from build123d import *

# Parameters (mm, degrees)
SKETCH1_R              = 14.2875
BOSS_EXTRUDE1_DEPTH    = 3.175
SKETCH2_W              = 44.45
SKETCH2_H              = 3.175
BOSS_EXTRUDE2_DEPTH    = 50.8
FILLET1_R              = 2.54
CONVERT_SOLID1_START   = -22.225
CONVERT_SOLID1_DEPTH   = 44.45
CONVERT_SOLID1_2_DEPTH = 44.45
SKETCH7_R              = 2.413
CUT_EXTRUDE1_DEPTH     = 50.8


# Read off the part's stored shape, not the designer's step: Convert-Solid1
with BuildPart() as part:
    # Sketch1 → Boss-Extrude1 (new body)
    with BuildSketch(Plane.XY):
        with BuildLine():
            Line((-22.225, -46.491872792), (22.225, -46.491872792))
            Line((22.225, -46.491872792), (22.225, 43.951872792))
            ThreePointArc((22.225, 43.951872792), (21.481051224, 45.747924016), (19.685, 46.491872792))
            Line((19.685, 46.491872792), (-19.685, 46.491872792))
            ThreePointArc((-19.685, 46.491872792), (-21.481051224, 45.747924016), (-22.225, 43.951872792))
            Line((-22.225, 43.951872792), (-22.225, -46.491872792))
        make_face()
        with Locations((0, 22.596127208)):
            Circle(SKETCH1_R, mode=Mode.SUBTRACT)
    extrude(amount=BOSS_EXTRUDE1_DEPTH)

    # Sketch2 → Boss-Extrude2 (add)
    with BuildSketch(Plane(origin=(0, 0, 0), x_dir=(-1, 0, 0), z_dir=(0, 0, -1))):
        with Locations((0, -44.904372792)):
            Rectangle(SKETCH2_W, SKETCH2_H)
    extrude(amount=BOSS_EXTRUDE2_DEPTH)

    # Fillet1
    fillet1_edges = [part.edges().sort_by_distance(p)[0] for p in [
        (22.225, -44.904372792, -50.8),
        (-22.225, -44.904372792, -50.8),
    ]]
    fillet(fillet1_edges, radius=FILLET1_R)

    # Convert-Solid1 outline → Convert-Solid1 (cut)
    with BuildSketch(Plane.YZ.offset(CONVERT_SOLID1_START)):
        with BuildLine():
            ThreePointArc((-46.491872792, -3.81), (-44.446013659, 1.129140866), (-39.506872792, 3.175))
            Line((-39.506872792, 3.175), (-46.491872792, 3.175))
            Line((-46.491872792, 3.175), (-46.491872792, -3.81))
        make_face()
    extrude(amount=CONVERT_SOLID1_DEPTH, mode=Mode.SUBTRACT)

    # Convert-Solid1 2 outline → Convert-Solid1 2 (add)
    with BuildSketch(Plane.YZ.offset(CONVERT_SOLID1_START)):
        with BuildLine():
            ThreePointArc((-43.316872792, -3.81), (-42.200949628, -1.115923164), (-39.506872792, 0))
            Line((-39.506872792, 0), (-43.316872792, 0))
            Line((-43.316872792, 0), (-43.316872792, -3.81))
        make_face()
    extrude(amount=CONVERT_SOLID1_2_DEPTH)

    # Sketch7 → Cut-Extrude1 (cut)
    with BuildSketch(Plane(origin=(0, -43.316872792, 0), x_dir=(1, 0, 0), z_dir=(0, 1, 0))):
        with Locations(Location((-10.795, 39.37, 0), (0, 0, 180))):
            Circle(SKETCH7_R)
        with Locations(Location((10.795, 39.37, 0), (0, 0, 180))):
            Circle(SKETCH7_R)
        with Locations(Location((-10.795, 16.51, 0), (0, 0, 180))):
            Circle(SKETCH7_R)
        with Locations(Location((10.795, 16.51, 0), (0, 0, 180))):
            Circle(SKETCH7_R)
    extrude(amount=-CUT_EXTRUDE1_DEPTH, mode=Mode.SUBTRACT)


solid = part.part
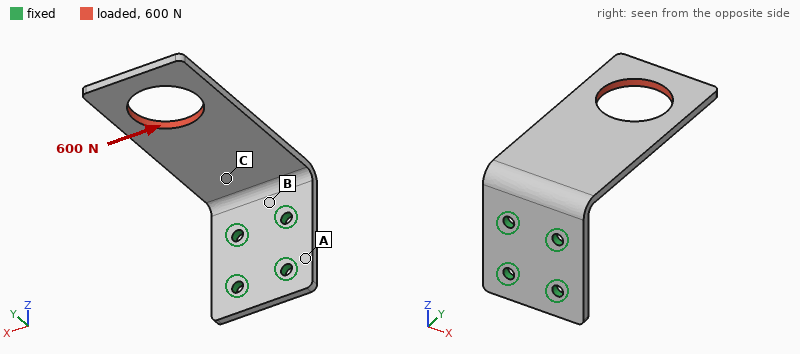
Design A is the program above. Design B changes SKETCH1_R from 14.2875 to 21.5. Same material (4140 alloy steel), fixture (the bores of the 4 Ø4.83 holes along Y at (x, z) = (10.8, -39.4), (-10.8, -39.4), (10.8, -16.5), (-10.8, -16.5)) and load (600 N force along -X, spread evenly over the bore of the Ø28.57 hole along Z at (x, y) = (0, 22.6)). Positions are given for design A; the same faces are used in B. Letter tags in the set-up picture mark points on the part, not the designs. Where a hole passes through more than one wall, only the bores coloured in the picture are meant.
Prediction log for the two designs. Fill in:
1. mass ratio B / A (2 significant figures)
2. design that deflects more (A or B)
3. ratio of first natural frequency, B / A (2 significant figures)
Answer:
0.85
B
1.2
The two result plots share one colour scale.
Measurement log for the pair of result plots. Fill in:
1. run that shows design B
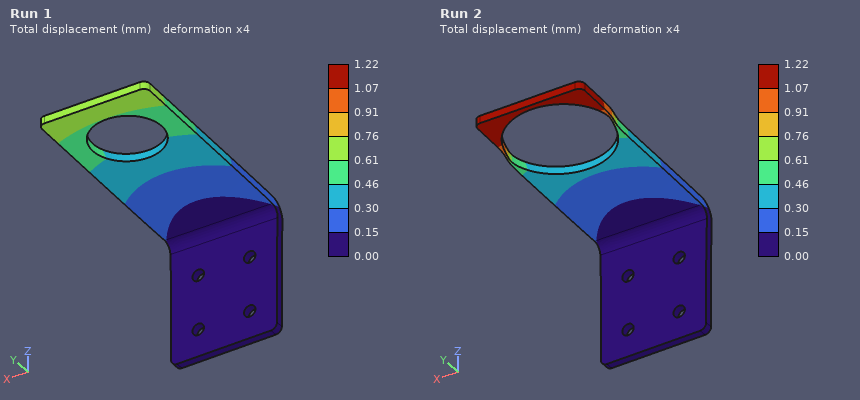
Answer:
Run 2
